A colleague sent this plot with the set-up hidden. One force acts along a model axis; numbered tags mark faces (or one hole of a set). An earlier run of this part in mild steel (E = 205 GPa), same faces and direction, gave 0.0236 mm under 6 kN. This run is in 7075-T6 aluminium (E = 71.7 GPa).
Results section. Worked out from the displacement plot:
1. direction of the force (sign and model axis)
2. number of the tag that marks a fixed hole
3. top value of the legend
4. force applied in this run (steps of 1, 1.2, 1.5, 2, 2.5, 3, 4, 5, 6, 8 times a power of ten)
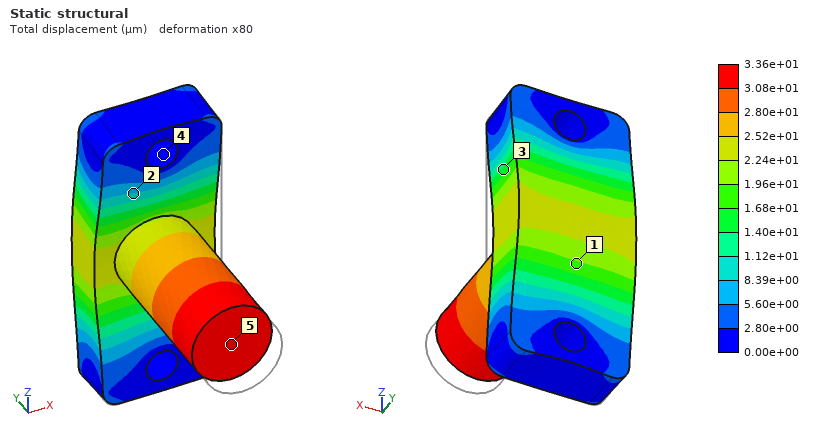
+Y
4
3.36e+01 µm
3 kN
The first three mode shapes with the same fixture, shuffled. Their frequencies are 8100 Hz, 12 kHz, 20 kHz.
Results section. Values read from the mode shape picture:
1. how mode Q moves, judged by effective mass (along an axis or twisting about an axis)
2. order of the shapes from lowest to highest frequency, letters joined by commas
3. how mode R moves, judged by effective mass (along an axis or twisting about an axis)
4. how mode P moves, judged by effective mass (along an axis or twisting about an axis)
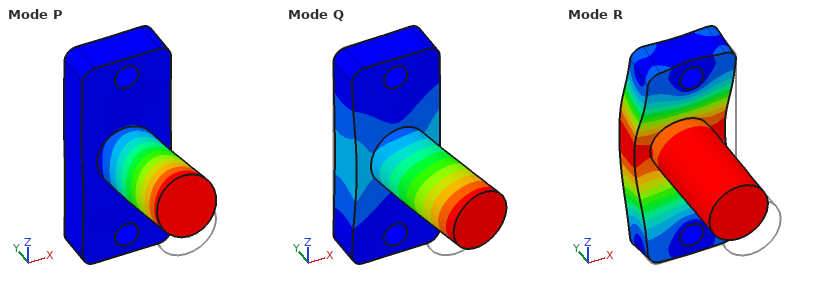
along X
Q, P, R
along Y
along Z
